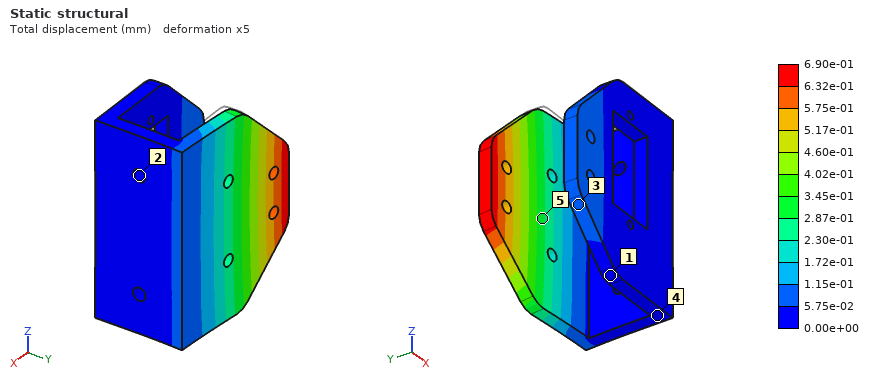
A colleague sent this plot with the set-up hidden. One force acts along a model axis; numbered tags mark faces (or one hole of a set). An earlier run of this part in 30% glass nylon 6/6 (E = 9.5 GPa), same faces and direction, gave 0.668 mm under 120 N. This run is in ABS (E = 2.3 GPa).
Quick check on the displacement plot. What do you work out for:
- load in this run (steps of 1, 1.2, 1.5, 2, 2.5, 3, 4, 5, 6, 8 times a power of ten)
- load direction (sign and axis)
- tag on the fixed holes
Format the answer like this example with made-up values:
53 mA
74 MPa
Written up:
30 N
+Y
2
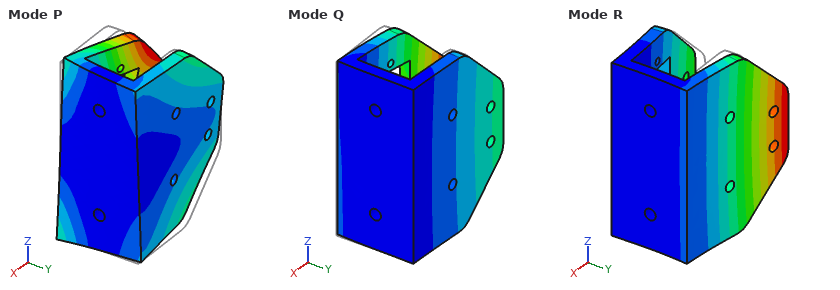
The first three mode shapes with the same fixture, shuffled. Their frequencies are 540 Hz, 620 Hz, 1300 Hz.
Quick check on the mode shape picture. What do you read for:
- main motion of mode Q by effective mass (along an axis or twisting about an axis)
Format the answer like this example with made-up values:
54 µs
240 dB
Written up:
along Y
